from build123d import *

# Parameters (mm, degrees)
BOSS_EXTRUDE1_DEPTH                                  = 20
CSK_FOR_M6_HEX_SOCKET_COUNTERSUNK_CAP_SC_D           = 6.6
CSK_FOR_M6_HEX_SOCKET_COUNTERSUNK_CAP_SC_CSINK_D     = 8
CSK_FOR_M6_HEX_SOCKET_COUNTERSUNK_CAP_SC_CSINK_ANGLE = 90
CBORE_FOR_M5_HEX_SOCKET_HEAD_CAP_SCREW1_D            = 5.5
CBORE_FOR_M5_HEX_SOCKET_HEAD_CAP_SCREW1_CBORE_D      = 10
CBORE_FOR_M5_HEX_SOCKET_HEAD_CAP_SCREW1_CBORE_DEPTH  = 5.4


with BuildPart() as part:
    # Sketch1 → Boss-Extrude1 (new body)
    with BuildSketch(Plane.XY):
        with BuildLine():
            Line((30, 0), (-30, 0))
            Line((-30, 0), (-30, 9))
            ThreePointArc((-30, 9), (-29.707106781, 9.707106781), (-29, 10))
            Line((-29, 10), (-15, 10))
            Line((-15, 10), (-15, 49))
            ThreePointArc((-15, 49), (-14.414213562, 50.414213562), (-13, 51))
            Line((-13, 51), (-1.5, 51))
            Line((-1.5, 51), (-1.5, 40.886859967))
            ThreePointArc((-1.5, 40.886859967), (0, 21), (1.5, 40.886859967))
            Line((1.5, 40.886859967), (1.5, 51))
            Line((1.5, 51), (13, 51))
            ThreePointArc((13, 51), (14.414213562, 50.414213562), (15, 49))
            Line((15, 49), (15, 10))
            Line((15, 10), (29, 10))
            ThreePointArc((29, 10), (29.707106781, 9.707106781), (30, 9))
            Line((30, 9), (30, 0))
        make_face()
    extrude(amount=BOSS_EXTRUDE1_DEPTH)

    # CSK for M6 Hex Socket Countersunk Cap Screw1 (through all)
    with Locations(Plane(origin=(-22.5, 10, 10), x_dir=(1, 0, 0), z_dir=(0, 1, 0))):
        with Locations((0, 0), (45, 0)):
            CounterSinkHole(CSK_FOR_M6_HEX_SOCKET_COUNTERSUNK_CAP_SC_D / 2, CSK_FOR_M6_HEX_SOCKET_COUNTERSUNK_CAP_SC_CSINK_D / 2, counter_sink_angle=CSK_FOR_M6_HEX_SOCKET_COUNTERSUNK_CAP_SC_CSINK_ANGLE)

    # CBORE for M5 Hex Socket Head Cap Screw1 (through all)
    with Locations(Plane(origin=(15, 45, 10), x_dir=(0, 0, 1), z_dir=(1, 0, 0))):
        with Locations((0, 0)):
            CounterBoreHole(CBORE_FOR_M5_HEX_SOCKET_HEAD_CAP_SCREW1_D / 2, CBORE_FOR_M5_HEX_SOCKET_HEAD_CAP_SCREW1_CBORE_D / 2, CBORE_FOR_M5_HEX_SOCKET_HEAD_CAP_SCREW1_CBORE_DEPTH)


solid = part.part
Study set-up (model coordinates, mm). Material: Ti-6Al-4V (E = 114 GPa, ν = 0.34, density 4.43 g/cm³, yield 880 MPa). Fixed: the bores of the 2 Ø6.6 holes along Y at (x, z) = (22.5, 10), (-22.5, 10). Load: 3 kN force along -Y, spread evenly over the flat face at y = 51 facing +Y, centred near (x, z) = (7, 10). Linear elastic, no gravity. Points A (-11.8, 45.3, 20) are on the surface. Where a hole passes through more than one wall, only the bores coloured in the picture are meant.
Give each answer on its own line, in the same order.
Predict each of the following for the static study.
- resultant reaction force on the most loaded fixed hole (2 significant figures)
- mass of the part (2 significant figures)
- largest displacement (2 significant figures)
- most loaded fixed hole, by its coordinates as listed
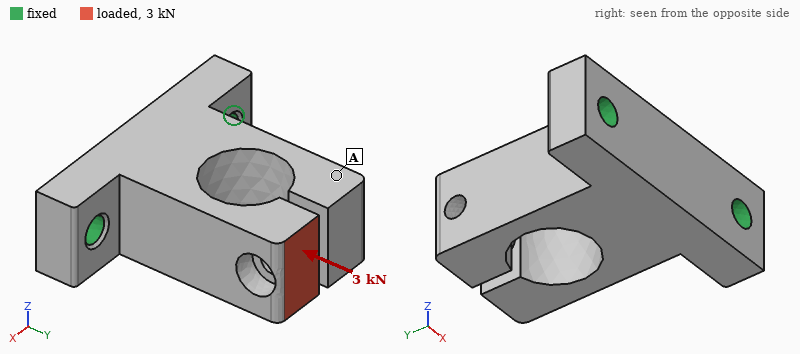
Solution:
2.2 kN
120 g
0.17 mm
(22.5, 10)
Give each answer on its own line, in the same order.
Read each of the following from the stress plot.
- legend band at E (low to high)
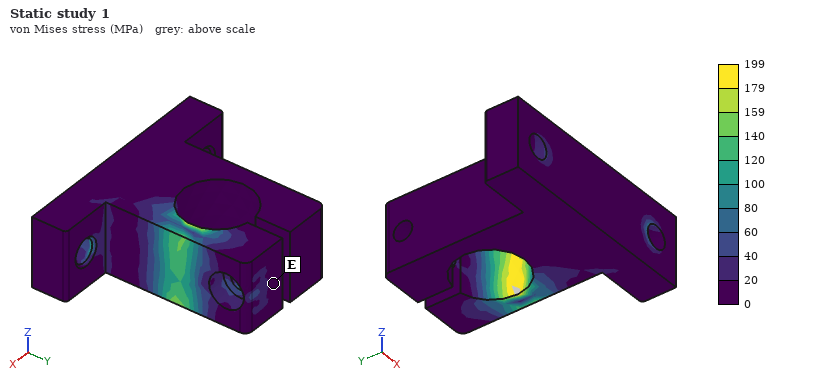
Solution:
0 to 20 MPa
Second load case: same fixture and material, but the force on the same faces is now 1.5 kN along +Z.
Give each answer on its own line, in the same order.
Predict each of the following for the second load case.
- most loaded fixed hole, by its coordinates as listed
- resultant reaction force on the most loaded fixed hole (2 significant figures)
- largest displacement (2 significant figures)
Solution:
(22.5, 10)
970 N
0.18 mm
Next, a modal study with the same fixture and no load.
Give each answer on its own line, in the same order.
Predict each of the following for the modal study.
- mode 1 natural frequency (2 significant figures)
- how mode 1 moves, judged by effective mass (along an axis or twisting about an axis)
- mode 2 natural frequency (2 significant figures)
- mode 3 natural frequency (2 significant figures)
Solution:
3600 Hz
along X
3700 Hz
3700 Hz
